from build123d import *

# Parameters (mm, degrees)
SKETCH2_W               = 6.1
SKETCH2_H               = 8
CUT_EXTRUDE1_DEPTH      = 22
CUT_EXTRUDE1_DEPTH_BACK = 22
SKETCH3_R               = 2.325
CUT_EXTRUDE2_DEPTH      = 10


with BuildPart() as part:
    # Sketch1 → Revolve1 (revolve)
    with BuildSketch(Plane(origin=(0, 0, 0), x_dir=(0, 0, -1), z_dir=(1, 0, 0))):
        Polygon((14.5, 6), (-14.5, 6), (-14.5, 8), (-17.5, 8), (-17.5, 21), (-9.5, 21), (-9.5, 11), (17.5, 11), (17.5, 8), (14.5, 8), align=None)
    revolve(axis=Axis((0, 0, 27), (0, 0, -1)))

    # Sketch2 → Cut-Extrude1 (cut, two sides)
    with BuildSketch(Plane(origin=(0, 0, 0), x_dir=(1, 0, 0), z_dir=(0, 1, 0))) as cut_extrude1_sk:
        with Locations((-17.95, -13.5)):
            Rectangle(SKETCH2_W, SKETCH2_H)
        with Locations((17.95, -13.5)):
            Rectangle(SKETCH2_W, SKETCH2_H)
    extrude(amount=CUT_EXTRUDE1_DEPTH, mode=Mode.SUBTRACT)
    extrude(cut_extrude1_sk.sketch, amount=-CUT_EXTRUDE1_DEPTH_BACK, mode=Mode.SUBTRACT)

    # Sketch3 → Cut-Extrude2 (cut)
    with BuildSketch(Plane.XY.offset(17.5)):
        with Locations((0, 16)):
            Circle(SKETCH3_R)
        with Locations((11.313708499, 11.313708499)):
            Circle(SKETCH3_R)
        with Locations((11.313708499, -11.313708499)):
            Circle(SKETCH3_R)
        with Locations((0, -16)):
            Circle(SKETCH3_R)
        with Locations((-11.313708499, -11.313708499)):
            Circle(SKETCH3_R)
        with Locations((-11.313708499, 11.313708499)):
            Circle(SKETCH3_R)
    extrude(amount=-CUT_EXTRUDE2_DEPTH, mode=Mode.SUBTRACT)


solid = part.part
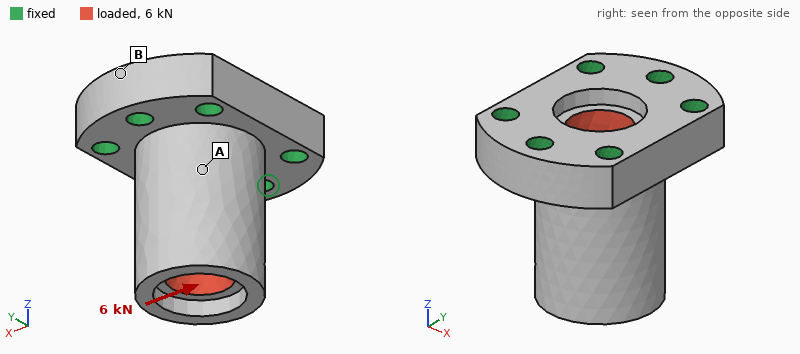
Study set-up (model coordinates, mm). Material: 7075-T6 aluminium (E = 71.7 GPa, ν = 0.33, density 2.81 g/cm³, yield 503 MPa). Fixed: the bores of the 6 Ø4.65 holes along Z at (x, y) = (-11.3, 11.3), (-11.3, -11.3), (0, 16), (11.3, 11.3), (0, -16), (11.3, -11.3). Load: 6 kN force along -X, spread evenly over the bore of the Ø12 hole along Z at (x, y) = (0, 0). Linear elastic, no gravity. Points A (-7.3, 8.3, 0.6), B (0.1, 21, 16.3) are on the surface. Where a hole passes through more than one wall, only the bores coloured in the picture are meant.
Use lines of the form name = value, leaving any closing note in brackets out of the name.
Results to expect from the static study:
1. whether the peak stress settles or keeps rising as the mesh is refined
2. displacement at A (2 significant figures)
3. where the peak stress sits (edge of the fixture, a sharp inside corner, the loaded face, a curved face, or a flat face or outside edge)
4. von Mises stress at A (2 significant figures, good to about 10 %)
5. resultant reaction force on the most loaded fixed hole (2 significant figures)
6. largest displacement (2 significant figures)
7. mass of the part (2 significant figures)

whether the peak stress settles or keeps rising as the mesh is refined = keeps rising
displacement at A = 22 µm
where the peak stress sits = edge of the fixture
von Mises stress at A = 25 MPa
resultant reaction force on the most loaded fixed hole = 2.3 kN
largest displacement = 51 µm
mass of the part = 39 g
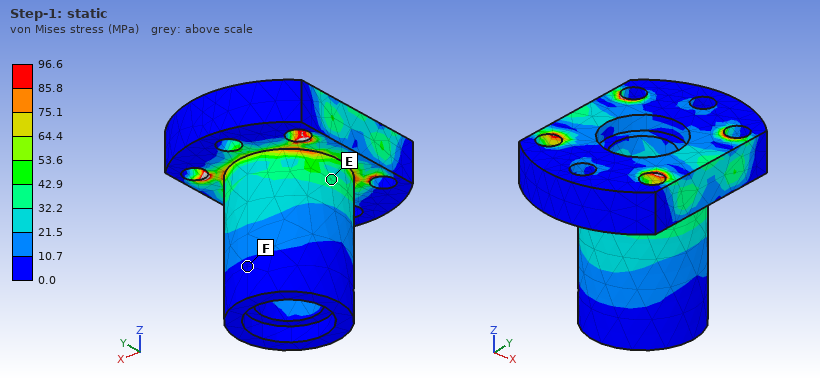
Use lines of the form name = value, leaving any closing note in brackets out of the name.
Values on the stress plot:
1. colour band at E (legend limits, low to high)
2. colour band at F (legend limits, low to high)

colour band at E = 32.2 to 42.9 MPa
colour band at F = 0.0 to 10.7 MPa
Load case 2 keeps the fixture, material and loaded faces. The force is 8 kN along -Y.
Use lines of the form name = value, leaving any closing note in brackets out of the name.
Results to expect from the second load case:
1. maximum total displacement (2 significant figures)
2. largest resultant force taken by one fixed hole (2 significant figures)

maximum total displacement = 56 µm
largest resultant force taken by one fixed hole = 2.6 kN
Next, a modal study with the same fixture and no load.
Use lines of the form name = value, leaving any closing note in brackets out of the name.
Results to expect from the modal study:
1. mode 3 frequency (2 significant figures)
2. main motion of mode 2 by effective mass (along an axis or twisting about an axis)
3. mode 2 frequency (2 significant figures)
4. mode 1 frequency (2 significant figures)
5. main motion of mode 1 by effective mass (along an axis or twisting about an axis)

mode 3 frequency = 26 kHz
main motion of mode 2 by effective mass = along Y
mode 2 frequency = 14 kHz
mode 1 frequency = 13 kHz
main motion of mode 1 by effective mass = along X
